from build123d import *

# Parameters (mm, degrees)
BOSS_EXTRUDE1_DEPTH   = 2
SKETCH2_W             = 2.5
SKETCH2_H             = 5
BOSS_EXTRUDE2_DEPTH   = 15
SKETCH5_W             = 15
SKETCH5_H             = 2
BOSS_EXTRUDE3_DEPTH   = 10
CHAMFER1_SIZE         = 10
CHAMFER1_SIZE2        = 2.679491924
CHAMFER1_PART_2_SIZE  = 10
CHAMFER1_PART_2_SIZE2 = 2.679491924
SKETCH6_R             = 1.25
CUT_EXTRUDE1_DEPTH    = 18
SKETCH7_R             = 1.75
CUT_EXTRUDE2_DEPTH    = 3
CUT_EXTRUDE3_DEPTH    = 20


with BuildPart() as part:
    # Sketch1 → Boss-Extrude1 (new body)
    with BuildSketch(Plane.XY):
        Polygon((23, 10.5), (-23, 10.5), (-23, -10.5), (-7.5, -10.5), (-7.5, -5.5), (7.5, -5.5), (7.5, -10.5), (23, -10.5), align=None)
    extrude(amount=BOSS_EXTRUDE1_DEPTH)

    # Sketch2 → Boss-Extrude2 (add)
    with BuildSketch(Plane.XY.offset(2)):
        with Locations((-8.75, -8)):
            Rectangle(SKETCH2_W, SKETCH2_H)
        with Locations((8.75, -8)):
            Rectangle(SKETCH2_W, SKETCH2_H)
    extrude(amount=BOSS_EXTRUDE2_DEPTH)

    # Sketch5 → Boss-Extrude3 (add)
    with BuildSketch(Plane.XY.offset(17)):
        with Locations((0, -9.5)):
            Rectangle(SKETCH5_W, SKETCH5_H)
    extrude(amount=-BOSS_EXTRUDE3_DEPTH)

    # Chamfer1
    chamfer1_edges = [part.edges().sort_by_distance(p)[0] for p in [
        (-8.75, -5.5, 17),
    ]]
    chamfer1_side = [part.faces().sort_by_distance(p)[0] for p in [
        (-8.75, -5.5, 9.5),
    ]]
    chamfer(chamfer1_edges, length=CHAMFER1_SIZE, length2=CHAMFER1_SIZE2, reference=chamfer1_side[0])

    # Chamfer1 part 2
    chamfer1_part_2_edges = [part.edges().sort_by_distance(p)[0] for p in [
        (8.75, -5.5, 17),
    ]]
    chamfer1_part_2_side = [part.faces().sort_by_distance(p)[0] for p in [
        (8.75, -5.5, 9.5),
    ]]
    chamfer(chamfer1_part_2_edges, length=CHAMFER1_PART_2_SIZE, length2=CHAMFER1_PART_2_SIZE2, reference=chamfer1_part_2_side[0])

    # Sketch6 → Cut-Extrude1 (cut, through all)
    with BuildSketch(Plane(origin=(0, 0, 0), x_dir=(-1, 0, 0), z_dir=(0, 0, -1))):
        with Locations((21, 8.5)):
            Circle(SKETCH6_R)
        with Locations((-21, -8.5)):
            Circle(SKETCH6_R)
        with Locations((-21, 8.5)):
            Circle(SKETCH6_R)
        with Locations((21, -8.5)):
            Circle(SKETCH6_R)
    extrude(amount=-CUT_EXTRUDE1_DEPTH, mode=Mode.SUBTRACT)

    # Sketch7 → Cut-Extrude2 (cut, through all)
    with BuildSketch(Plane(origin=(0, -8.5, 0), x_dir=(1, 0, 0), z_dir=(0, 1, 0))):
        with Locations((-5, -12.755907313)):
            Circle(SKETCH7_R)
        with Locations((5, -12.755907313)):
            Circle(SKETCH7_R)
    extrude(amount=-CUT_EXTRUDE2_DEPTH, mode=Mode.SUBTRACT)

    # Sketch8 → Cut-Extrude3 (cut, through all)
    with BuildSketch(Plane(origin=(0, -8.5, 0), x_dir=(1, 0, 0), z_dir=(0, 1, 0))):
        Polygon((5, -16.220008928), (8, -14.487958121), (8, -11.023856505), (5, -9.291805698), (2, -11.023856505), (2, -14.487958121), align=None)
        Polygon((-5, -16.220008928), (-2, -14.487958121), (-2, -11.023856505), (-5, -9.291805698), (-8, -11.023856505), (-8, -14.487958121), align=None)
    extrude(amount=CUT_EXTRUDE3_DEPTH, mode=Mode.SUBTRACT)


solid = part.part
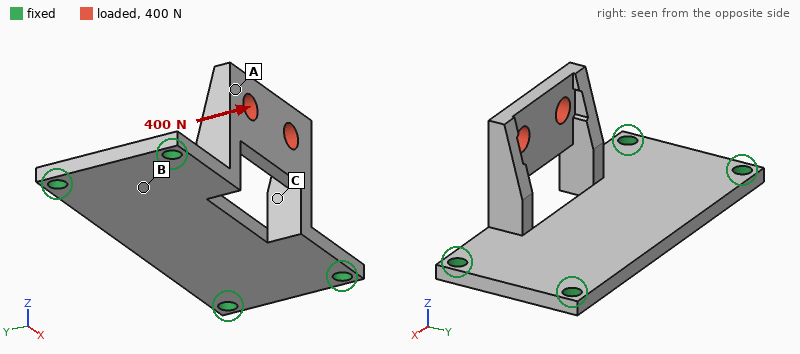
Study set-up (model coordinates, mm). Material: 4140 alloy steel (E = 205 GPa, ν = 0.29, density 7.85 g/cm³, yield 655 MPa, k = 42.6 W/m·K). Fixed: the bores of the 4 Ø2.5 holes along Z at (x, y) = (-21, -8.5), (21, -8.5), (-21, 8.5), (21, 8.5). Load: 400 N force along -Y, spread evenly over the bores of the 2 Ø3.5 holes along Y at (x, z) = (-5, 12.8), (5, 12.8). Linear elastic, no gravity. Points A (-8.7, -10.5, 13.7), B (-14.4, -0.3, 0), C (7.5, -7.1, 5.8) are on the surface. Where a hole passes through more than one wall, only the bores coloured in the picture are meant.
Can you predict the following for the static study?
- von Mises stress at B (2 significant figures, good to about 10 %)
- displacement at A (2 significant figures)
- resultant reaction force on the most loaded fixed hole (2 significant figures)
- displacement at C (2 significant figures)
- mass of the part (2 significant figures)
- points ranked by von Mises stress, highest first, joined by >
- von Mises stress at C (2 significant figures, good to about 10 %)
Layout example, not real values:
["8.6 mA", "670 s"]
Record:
["66 MPa", "0.14 mm", "250 N", "0.049 mm", "18 g", "C > B > A", "130 MPa"]
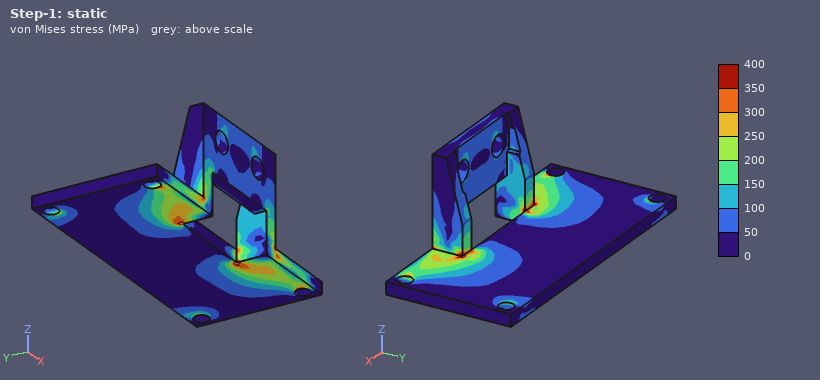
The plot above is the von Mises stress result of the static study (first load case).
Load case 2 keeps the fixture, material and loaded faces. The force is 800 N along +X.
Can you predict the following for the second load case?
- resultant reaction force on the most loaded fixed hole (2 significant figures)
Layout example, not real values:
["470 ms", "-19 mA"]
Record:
["400 N"]
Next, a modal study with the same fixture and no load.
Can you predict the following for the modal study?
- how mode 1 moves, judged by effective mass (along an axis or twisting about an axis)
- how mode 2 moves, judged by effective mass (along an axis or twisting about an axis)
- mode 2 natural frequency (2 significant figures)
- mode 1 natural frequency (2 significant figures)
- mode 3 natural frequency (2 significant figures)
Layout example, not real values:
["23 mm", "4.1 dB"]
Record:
["along Y", "along Z", "5900 Hz", "4700 Hz", "8900 Hz"]
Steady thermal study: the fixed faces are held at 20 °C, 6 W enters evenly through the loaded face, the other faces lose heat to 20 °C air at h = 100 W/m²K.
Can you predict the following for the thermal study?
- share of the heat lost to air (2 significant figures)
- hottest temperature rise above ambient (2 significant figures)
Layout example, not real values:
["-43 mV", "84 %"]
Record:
["65 %", "58 K"]
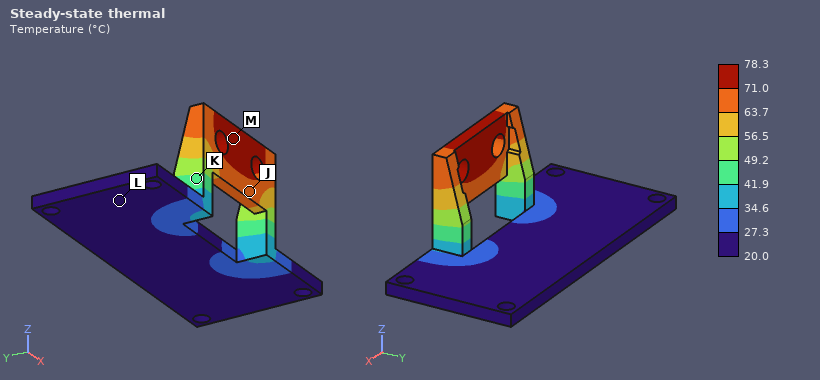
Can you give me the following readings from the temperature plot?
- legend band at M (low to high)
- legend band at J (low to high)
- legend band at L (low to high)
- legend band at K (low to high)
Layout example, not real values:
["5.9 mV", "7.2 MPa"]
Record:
["71.0 to 78.3 °C", "63.7 to 71.0 °C", "20.0 to 27.3 °C", "41.9 to 49.2 °C"]
